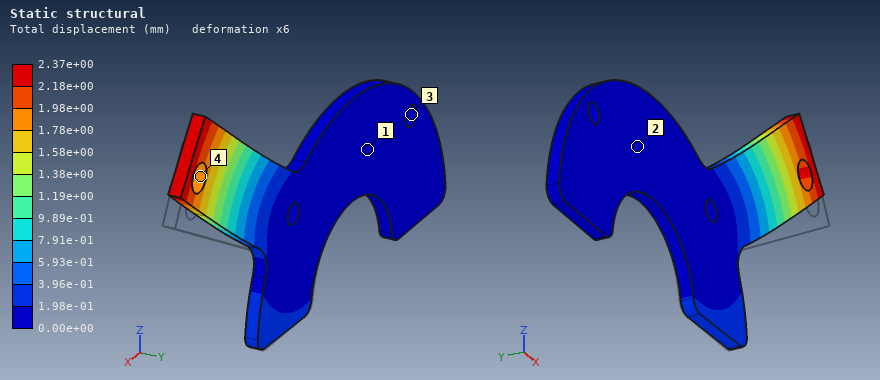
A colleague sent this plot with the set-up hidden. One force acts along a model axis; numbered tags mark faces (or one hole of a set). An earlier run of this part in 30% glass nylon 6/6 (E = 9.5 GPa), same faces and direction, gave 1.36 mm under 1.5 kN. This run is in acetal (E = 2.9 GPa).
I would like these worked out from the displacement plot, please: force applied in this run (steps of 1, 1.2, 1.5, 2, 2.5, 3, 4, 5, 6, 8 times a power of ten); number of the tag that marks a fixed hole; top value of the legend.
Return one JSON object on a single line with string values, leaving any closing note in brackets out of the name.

{"force applied in this run": "800 N", "number of the tag that marks a fixed hole": "3", "top value of the legend": "2.37e+00 mm"}
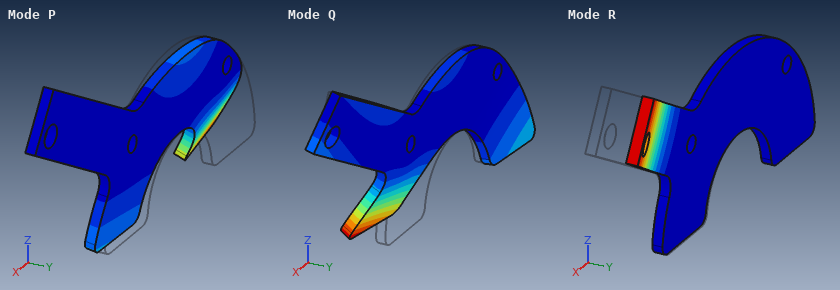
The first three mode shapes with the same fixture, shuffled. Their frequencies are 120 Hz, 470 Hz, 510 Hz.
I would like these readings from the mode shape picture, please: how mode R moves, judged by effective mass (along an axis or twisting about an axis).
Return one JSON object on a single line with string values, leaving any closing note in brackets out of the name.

{"how mode R moves, judged by effective mass": "along Y"}
